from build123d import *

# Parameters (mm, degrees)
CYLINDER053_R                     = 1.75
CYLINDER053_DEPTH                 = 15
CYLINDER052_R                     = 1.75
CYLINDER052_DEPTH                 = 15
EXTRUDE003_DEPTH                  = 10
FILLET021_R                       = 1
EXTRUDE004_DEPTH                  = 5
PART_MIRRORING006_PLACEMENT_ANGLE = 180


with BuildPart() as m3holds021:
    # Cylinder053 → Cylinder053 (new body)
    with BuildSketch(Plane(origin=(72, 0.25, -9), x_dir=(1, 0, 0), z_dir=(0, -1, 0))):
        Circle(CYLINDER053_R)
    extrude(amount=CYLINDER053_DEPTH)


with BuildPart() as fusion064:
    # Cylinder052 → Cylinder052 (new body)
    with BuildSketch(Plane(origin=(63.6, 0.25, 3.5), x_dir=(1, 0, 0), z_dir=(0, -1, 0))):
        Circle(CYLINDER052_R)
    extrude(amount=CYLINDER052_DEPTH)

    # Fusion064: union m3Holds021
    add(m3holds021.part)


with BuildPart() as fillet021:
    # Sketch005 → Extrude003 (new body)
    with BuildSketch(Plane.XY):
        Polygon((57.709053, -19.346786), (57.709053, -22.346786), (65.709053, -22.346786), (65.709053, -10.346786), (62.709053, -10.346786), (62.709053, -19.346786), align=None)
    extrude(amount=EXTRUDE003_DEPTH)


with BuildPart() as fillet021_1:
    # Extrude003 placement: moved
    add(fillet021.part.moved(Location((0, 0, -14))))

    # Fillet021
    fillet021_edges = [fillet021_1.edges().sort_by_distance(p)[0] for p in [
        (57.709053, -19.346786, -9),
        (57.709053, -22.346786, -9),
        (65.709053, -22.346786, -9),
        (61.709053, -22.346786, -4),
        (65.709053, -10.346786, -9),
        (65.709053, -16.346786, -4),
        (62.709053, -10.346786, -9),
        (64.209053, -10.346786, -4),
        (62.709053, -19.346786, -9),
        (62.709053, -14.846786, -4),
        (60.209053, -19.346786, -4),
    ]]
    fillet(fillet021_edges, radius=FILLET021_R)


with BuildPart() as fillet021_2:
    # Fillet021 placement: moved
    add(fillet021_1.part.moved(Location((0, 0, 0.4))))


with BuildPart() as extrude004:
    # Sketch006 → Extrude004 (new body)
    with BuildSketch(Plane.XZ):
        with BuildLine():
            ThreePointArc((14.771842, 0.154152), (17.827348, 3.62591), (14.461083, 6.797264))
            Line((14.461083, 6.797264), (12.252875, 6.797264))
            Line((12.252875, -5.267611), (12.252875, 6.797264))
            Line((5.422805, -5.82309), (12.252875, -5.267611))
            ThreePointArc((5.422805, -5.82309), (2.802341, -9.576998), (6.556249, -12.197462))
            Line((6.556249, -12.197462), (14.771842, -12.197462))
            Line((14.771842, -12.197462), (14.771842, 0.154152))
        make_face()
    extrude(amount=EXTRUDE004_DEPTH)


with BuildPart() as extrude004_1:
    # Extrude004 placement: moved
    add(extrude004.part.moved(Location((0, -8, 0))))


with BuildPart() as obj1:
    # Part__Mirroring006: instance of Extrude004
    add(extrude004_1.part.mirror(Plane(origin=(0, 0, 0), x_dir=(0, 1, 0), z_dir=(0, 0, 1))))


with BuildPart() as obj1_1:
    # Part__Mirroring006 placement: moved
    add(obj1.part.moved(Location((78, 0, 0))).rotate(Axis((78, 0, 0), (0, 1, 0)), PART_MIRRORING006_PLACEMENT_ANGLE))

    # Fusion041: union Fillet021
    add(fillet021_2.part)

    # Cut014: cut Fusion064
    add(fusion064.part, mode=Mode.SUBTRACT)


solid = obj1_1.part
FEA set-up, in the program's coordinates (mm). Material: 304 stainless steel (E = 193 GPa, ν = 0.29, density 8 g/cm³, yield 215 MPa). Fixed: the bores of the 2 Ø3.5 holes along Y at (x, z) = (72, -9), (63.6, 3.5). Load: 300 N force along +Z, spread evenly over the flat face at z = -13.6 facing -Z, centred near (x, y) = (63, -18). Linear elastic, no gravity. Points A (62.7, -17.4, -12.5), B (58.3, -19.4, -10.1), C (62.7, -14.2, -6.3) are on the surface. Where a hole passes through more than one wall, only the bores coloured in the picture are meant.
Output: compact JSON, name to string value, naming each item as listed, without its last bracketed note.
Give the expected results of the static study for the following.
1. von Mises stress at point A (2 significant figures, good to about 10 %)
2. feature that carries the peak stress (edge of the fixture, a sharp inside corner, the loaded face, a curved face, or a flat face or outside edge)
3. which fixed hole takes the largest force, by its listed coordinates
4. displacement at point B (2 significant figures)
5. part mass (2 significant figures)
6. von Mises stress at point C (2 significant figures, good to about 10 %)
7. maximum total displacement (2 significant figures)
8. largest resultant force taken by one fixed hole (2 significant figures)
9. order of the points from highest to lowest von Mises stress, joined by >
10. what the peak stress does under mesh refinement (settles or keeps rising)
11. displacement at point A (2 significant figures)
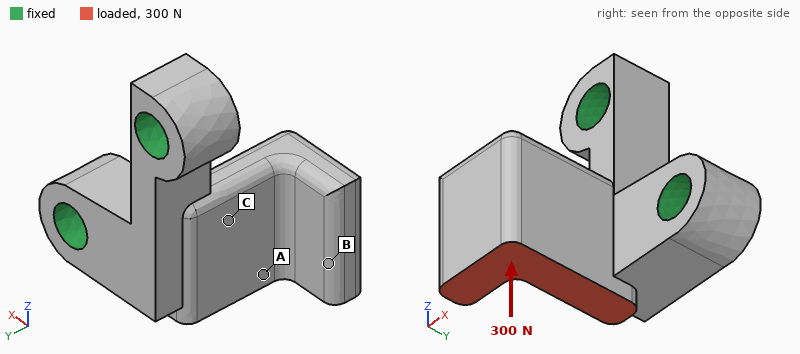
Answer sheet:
{"von Mises stress at point A": "24 MPa", "feature that carries the peak stress": "a sharp inside corner", "which fixed hole takes the largest force, by its listed coordinates": "(63.6, 3.5)", "displacement at point B": "9.4 µm", "part mass": "7.6 g", "von Mises stress at point C": "38 MPa", "maximum total displacement": "12 µm", "largest resultant force taken by one fixed hole": "290 N", "order of the points from highest to lowest von Mises stress, joined by >": "C > A > B", "what the peak stress does under mesh refinement": "keeps rising", "displacement at point A": "6.4 µm"}
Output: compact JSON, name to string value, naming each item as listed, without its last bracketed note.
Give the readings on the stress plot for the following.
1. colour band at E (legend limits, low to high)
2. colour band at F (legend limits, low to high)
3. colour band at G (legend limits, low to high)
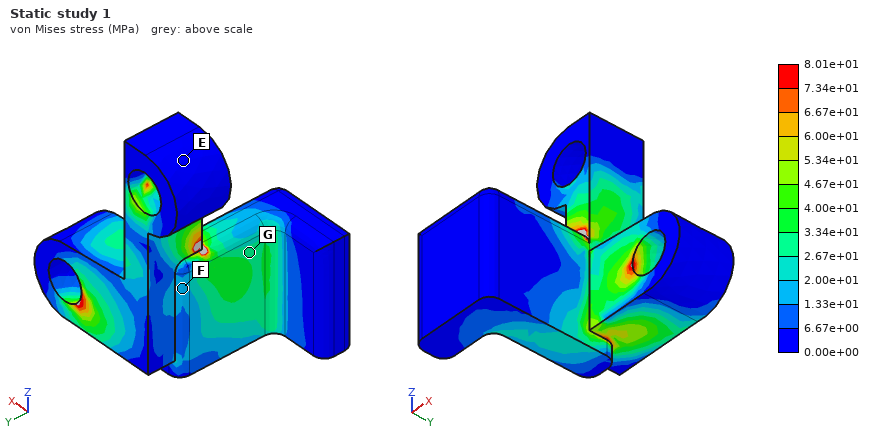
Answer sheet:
{"colour band at E": "0.00e+00 to 6.67e+00 MPa", "colour band at F": "1.33e+01 to 2.00e+01 MPa", "colour band at G": "2.67e+01 to 3.34e+01 MPa"}
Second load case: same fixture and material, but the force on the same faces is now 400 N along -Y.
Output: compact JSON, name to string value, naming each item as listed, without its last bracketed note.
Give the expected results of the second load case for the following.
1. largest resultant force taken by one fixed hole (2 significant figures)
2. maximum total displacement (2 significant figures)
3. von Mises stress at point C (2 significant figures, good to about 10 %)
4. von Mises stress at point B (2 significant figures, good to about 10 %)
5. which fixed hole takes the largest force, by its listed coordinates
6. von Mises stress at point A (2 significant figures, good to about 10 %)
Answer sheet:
{"largest resultant force taken by one fixed hole": "420 N", "maximum total displacement": "31 µm", "von Mises stress at point C": "37 MPa", "von Mises stress at point B": "18 MPa", "which fixed hole takes the largest force, by its listed coordinates": "(72, -9)", "von Mises stress at point A": "65 MPa"}
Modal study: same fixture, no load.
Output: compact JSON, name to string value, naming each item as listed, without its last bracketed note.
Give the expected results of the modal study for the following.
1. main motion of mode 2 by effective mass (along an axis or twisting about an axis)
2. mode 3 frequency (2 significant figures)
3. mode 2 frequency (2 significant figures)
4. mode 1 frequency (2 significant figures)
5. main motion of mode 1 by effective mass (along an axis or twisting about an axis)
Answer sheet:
{"main motion of mode 2 by effective mass": "along Z", "mode 3 frequency": "25 kHz", "mode 2 frequency": "16 kHz", "mode 1 frequency": "9100 Hz", "main motion of mode 1 by effective mass": "along X"}
